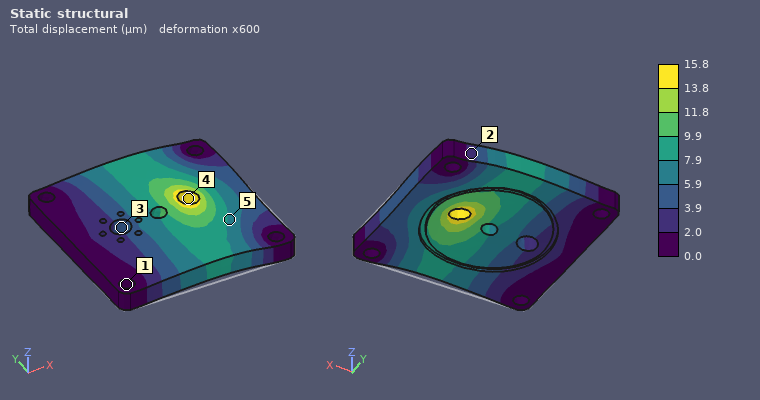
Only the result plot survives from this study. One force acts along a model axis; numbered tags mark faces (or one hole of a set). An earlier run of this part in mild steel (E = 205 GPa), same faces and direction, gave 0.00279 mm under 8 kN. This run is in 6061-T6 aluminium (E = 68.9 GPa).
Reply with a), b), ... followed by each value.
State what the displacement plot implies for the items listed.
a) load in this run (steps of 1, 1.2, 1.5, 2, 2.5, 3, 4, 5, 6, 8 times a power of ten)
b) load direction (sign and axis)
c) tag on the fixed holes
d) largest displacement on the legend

a) 15 kN
b) +Y
c) 1
d) 15.8 µm
